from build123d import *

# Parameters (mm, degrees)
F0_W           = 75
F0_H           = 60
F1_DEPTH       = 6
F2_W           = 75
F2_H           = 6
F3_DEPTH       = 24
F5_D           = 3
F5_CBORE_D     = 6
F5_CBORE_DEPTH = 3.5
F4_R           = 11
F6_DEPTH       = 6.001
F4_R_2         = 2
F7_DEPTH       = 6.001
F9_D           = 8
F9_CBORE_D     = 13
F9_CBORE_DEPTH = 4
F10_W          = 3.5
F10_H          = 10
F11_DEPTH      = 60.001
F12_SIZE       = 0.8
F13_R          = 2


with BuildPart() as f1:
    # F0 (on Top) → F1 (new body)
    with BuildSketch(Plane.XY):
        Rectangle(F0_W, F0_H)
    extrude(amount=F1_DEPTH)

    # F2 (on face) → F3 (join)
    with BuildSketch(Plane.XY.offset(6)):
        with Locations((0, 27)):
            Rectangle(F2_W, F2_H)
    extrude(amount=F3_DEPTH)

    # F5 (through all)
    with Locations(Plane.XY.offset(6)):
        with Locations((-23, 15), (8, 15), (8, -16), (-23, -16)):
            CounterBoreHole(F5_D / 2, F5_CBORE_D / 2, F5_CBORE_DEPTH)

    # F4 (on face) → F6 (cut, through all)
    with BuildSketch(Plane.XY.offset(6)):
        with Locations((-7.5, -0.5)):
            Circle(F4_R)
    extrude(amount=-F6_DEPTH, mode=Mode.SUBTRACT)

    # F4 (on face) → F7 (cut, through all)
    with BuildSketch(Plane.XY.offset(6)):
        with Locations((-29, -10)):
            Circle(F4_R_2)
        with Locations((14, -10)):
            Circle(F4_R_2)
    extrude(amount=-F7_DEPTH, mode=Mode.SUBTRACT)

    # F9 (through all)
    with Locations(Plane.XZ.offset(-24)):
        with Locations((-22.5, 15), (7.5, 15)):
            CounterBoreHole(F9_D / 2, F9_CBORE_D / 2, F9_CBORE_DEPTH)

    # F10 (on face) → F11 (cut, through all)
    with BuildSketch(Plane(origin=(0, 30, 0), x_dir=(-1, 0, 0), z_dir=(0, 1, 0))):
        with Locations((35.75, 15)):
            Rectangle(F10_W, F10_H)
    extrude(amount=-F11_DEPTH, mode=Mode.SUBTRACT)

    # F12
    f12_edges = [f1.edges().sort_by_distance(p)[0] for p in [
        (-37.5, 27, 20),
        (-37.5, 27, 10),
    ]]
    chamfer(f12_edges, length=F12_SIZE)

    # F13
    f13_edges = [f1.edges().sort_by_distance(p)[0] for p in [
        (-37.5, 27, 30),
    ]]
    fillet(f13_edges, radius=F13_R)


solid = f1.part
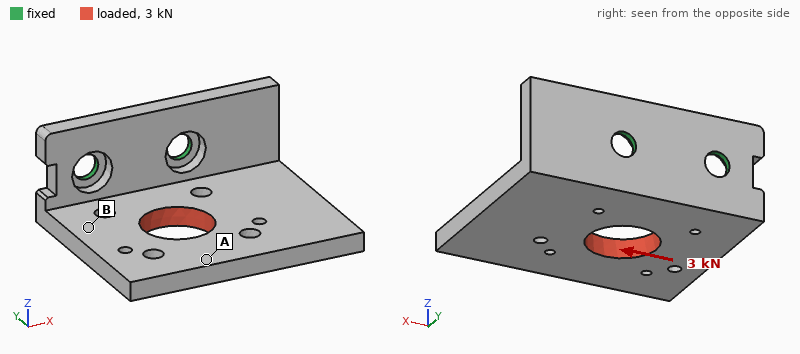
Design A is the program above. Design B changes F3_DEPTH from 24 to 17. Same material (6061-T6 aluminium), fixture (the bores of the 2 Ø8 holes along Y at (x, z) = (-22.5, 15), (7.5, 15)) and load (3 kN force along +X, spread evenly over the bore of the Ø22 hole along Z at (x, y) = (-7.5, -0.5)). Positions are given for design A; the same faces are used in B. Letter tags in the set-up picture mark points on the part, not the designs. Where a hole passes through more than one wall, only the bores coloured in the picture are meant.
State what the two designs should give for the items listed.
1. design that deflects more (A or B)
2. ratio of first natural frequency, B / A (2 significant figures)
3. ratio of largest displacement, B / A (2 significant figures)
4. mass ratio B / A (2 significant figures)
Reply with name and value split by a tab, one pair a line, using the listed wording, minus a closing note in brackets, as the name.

design that deflects more	B
ratio of first natural frequency, B / A	0.97
ratio of largest displacement, B / A	1.1
mass ratio B / A	0.91
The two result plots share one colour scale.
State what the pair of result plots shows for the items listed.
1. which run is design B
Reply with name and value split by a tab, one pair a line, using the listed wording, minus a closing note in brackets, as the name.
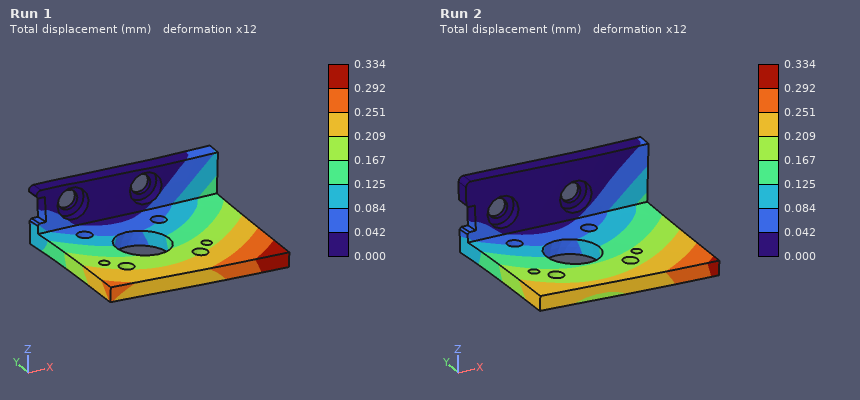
which run is design B	Run 1
